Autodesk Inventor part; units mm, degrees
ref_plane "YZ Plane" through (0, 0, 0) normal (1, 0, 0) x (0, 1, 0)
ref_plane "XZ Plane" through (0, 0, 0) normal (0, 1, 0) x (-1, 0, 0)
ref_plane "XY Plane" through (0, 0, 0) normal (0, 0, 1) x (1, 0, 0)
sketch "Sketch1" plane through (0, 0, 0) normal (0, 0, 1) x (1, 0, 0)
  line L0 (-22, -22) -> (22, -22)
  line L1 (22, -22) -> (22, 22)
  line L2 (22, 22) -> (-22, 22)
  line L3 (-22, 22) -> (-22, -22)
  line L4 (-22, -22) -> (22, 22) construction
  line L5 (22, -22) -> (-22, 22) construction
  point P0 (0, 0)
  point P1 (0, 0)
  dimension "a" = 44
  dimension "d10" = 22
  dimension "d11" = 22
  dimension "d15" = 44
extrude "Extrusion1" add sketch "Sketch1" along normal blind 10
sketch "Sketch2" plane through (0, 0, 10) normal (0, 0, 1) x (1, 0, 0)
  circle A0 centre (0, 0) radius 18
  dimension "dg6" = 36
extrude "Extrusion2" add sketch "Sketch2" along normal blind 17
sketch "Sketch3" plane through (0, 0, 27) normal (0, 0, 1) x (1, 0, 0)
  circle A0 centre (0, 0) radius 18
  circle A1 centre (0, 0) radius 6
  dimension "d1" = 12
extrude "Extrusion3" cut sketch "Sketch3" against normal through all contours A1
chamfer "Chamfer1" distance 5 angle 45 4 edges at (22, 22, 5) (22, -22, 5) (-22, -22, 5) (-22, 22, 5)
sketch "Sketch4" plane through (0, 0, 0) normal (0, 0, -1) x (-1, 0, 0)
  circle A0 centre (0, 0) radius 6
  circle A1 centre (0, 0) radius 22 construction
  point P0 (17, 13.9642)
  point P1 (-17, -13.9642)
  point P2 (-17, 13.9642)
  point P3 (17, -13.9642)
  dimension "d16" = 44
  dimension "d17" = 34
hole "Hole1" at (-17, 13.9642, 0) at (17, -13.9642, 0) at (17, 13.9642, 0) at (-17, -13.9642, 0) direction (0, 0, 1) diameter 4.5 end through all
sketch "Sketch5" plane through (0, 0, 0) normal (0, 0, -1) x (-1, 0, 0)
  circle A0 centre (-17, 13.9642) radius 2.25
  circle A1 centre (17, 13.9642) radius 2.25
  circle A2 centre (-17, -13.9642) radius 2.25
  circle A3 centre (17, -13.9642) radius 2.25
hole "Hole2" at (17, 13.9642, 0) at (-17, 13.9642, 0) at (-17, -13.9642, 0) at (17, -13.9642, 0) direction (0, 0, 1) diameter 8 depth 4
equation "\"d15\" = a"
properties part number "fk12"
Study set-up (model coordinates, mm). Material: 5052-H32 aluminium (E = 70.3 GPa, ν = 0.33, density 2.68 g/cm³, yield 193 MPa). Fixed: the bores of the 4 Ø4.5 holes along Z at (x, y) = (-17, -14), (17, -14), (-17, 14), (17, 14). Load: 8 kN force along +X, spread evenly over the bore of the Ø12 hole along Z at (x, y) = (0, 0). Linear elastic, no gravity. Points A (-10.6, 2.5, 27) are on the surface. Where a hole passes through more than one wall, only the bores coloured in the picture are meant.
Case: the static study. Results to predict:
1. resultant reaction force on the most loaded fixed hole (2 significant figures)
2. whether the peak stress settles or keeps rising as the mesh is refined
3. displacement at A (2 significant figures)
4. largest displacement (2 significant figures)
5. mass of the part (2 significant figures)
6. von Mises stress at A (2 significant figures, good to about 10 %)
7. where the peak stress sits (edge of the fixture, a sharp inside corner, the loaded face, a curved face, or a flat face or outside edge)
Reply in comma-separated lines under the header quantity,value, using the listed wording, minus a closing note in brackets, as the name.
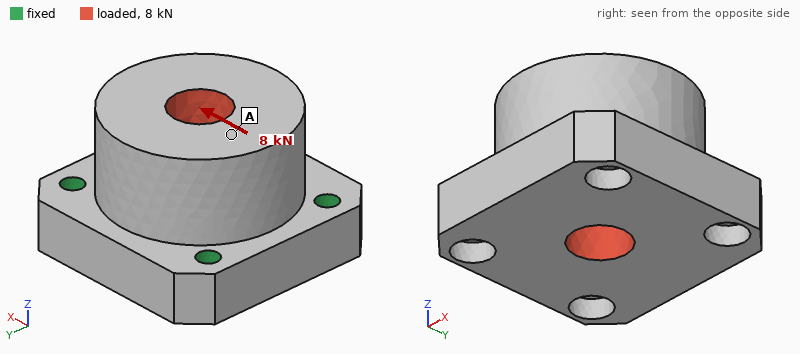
quantity,value
resultant reaction force on the most loaded fixed hole,2.2 kN
whether the peak stress settles or keeps rising as the mesh is refined,keeps rising
displacement at A,9.9 µm
largest displacement,10 µm
mass of the part,86 g
von Mises stress at A,8.1 MPa
where the peak stress sits,edge of the fixture
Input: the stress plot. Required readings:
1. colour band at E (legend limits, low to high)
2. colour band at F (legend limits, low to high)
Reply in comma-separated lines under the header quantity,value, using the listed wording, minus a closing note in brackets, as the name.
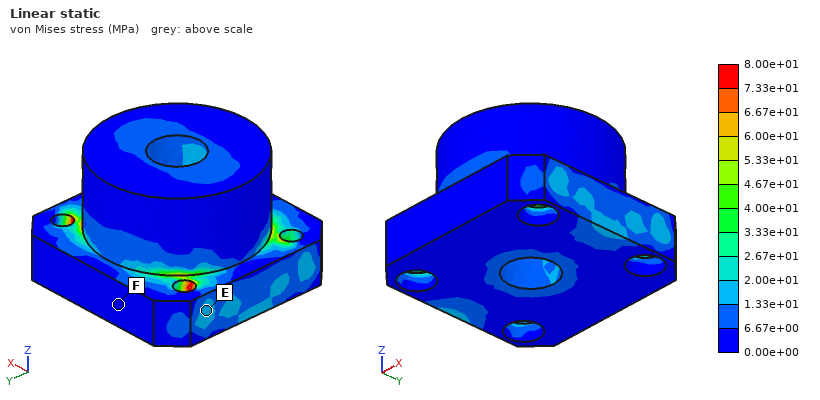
quantity,value
colour band at E,1.33e+01 to 2.00e+01 MPa
colour band at F,0.00e+00 to 6.67e+00 MPa
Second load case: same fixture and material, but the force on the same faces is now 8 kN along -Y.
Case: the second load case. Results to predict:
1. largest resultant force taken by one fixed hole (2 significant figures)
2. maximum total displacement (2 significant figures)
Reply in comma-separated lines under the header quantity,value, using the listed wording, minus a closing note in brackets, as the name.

quantity,value
largest resultant force taken by one fixed hole,2.3 kN
maximum total displacement,13 µm
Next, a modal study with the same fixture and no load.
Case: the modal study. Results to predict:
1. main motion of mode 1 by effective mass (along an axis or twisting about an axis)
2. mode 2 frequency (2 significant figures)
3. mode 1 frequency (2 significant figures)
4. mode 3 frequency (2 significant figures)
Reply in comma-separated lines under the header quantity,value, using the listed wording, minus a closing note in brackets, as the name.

quantity,value
main motion of mode 1 by effective mass,along Y
mode 2 frequency,20 kHz
mode 1 frequency,17 kHz
mode 3 frequency,20 kHz
